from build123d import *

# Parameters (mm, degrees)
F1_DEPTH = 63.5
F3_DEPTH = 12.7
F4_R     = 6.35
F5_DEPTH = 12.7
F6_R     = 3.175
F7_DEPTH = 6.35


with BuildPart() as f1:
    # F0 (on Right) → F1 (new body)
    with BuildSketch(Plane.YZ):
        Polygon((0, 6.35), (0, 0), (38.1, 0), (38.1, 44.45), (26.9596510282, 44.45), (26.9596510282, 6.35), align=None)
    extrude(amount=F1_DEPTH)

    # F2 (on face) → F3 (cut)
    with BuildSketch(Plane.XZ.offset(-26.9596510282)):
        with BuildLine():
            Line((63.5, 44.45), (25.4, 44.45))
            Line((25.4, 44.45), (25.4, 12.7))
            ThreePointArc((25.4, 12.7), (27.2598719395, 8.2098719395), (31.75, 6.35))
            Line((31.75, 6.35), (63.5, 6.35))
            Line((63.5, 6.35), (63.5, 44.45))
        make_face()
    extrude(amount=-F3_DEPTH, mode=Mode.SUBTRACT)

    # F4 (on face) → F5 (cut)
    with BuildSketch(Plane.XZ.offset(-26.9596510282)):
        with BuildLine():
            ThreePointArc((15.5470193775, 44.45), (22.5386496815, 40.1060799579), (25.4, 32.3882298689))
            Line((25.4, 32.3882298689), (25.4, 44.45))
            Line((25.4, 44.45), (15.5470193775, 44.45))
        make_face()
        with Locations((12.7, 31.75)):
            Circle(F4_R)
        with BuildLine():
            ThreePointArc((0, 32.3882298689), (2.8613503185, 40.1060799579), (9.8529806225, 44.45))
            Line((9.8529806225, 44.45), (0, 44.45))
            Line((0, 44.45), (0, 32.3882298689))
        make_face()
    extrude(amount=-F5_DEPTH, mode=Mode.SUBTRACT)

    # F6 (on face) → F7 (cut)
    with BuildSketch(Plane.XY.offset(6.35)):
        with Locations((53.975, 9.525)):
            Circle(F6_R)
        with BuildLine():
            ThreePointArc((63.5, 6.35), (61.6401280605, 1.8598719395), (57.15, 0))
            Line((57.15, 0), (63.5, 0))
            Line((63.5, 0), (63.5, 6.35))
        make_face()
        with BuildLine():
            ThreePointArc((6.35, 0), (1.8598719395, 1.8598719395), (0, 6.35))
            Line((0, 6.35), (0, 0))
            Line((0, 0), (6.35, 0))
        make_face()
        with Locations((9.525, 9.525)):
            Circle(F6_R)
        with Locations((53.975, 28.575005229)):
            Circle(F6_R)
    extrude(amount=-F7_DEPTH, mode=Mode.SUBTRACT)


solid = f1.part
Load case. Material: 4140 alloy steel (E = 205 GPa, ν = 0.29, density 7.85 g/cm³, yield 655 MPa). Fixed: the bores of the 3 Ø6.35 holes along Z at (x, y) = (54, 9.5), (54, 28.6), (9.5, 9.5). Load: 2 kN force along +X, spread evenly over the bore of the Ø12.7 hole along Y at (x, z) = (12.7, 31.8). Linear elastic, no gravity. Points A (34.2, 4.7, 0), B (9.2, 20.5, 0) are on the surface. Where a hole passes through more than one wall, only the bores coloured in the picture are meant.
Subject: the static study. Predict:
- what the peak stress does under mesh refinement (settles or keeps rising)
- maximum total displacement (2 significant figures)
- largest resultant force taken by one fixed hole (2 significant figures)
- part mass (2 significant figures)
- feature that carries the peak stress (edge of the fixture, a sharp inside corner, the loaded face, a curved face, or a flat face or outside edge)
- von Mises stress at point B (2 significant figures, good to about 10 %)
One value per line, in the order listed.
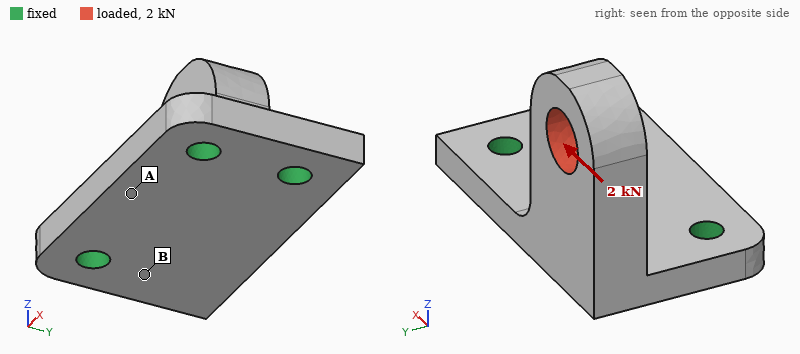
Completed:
keeps rising
0.10 mm
1.5 kN
180 g
edge of the fixture
89 MPa
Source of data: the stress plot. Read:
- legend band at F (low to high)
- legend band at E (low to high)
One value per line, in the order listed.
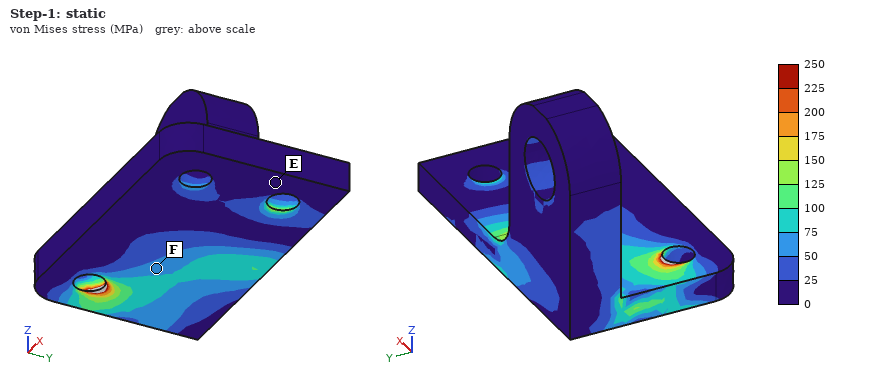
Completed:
50 to 75 MPa
0 to 25 MPa
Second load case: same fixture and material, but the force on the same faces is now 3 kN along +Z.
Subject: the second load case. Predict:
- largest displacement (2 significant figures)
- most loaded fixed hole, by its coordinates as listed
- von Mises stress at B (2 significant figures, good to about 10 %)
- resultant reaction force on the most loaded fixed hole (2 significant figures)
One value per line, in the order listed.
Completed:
0.15 mm
(9.5, 9.5)
110 MPa
2.4 kN
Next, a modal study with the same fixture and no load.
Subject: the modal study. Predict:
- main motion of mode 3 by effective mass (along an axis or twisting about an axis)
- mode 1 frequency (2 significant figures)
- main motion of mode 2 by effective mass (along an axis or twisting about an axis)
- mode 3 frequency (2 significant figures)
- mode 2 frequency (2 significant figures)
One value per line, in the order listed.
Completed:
along Z
2300 Hz
along X
7100 Hz
4400 Hz
